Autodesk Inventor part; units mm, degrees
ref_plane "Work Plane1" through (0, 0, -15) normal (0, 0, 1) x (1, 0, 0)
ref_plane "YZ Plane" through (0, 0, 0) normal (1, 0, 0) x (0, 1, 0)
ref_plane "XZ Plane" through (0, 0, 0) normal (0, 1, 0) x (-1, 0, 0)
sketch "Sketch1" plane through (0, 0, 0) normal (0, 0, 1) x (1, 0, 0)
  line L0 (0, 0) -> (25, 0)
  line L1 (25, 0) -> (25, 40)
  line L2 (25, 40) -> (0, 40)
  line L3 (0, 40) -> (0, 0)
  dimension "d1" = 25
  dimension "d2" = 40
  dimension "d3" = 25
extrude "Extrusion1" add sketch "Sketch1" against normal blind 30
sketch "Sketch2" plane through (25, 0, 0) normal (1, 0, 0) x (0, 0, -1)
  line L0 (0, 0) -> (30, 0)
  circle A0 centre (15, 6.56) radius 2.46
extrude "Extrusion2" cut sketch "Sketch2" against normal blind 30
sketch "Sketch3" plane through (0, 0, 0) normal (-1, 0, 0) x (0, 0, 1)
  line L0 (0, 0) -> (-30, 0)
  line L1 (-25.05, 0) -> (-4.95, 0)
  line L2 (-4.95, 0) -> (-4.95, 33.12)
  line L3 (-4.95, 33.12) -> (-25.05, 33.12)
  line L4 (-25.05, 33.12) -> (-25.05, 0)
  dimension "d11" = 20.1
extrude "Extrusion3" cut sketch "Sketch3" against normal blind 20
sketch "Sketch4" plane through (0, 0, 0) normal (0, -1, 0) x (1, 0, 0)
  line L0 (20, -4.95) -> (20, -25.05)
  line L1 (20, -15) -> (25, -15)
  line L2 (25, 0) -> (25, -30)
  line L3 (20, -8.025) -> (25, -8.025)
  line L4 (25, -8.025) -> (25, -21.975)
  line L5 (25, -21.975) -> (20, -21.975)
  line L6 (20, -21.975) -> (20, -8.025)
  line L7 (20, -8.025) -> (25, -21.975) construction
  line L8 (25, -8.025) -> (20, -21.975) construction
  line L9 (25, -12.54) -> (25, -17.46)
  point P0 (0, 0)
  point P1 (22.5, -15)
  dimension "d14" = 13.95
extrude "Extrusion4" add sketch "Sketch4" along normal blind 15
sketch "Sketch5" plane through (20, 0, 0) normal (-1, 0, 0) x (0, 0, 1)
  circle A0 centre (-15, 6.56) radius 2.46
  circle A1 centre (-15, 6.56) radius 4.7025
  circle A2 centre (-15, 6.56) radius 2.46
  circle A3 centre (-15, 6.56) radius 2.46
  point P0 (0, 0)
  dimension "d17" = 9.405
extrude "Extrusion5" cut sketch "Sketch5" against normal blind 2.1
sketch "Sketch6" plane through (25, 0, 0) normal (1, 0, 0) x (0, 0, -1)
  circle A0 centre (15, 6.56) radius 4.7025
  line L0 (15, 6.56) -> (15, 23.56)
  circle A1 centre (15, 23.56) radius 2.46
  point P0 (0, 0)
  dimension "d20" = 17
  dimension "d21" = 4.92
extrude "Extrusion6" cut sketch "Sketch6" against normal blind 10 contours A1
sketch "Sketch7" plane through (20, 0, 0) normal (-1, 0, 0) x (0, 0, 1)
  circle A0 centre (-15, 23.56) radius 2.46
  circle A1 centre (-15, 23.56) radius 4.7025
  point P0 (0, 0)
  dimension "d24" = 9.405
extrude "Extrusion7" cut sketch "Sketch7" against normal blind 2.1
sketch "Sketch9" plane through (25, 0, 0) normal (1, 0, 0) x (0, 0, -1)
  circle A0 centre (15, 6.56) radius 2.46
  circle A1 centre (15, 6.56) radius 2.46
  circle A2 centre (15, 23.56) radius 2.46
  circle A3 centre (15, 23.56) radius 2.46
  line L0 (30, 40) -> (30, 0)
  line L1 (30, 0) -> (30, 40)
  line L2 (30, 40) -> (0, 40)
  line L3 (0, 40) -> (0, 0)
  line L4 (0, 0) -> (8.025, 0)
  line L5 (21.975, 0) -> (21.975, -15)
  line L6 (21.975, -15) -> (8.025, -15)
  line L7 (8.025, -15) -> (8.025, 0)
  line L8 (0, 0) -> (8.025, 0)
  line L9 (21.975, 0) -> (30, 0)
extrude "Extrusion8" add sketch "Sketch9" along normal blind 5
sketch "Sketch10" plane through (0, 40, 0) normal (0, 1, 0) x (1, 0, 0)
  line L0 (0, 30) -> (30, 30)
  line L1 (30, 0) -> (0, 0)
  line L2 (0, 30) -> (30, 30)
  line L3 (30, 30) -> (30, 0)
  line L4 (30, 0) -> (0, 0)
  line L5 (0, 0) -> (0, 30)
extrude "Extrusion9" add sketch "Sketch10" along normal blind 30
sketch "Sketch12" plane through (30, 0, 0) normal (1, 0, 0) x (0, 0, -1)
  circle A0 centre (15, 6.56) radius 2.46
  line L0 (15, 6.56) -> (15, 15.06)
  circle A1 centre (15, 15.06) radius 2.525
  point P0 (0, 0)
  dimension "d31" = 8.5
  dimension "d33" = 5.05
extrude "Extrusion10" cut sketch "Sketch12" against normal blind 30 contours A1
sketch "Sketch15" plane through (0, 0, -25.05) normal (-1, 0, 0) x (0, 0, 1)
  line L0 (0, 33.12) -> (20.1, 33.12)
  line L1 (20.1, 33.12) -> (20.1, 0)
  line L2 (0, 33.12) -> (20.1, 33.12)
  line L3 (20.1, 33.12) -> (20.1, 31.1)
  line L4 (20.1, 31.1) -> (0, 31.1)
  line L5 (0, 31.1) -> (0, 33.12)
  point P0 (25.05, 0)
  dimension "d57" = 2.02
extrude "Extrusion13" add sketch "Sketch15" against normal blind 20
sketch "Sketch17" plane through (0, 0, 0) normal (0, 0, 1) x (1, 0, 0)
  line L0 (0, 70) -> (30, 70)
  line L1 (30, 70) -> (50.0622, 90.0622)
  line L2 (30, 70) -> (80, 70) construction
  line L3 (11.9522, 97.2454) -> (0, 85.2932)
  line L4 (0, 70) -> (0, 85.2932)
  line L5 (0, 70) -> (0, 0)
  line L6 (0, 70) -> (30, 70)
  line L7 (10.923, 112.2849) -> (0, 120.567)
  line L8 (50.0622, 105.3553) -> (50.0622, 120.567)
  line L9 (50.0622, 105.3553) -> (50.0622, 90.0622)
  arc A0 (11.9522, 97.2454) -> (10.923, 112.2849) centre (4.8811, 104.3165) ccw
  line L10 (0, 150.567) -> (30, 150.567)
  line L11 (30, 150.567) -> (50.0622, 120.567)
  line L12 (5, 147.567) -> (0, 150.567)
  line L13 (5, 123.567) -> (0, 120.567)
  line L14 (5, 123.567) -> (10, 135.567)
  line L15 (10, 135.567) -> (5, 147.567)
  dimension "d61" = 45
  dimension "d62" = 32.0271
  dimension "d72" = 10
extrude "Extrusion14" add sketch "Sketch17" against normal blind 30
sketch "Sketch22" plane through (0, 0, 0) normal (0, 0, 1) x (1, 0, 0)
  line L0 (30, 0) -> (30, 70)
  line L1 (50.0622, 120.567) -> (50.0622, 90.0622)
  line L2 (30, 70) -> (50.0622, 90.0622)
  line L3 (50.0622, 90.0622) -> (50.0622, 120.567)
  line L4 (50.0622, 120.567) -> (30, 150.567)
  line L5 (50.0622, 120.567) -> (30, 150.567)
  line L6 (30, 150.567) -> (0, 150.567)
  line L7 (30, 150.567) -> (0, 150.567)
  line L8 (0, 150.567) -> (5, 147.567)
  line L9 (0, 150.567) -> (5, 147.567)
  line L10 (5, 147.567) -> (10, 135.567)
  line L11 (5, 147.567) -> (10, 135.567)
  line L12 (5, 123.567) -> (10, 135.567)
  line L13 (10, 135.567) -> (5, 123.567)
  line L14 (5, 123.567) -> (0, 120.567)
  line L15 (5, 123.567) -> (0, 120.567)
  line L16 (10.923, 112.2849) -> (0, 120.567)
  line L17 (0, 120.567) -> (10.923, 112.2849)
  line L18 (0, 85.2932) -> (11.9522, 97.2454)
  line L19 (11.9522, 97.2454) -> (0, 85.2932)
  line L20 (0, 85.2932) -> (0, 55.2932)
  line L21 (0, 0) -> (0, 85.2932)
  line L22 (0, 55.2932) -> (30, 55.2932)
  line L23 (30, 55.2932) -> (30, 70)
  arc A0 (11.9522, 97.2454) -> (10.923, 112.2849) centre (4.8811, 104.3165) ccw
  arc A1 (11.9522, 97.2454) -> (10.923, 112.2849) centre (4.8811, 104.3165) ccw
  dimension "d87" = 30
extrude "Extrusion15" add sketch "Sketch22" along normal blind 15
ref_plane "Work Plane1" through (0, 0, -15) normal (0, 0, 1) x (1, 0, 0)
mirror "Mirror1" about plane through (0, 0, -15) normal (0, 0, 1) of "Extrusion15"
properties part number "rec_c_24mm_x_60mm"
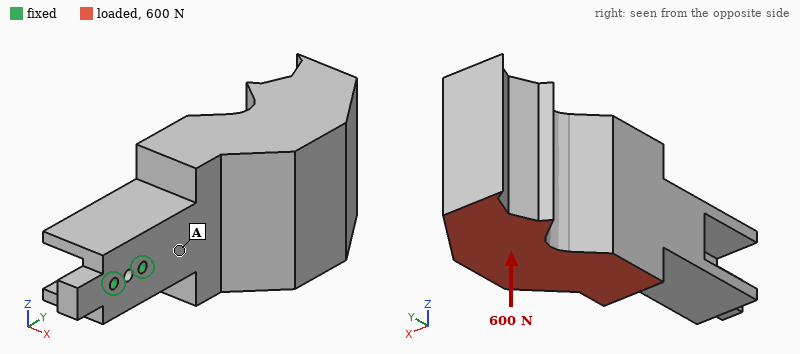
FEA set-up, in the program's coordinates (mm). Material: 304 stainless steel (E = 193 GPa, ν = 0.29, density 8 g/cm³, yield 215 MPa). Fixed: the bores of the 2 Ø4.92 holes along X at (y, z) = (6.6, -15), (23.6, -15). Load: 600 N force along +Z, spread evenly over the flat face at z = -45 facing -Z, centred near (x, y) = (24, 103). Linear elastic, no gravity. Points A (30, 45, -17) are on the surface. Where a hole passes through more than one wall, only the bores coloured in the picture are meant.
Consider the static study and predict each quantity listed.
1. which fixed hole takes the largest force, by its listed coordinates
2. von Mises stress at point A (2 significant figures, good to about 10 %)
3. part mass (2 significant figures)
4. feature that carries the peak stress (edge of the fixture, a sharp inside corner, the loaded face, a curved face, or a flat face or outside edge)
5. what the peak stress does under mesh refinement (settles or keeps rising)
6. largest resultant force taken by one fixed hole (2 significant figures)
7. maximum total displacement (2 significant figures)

(23.6, -15)
5.9 MPa
2.0 kg
edge of the fixture
keeps rising
2.6 kN
45 µm
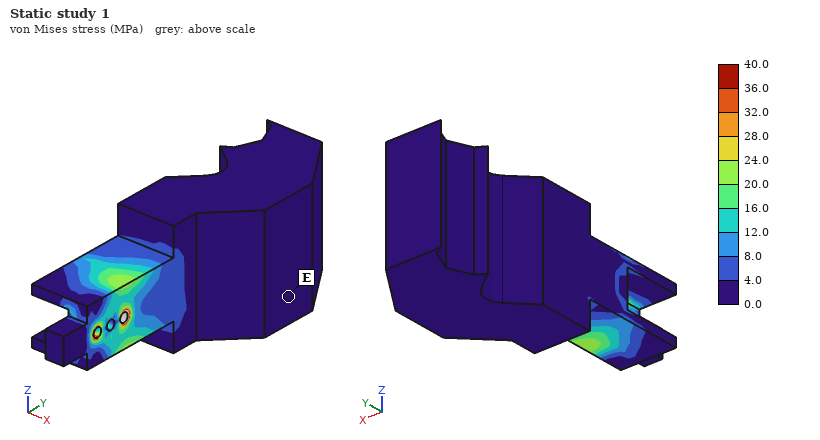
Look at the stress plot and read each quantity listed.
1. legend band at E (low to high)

0.0 to 4.0 MPa
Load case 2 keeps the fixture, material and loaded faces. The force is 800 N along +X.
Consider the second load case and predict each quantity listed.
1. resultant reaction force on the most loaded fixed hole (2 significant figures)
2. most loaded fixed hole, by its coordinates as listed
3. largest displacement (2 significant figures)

3.3 kN
(23.6, -15)
95 µm
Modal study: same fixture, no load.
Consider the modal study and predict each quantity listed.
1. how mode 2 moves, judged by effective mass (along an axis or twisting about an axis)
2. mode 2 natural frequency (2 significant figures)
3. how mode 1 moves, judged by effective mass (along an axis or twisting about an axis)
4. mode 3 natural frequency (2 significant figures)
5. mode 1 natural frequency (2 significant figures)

along Z
540 Hz
along X
1300 Hz
470 Hz
